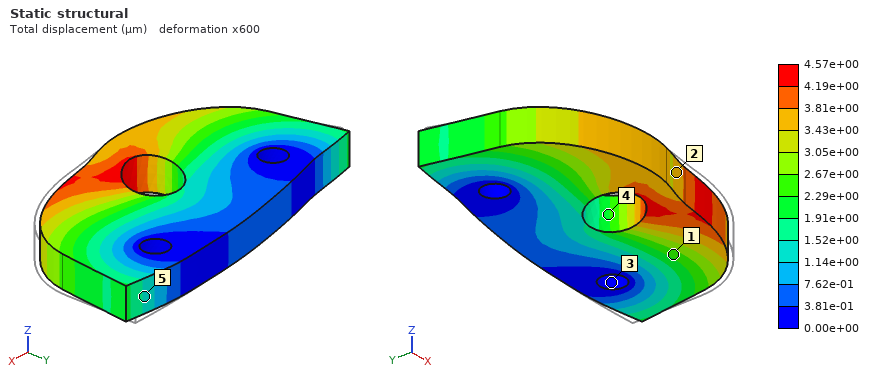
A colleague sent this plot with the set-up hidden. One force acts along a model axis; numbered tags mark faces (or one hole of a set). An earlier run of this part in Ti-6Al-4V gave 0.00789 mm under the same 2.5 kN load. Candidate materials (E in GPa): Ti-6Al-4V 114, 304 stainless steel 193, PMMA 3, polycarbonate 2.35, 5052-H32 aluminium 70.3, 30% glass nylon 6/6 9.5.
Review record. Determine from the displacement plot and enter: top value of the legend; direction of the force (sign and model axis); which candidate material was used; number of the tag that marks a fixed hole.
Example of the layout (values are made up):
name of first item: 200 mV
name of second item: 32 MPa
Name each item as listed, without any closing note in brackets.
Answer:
top value of the legend: 4.57e+00 µm
direction of the force: -X
which candidate material was used: 304 stainless steel
number of the tag that marks a fixed hole: 3
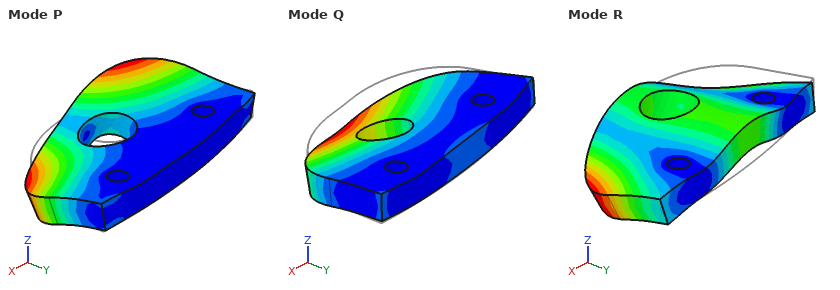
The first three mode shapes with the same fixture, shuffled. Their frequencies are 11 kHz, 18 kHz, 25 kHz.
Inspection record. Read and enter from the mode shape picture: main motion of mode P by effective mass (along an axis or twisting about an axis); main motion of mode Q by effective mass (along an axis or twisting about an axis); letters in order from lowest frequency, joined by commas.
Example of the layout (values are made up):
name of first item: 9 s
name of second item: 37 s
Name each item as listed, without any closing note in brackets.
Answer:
main motion of mode P by effective mass: twisting about Y
main motion of mode Q by effective mass: along Z
letters in order from lowest frequency, joined by commas: Q, P, R
